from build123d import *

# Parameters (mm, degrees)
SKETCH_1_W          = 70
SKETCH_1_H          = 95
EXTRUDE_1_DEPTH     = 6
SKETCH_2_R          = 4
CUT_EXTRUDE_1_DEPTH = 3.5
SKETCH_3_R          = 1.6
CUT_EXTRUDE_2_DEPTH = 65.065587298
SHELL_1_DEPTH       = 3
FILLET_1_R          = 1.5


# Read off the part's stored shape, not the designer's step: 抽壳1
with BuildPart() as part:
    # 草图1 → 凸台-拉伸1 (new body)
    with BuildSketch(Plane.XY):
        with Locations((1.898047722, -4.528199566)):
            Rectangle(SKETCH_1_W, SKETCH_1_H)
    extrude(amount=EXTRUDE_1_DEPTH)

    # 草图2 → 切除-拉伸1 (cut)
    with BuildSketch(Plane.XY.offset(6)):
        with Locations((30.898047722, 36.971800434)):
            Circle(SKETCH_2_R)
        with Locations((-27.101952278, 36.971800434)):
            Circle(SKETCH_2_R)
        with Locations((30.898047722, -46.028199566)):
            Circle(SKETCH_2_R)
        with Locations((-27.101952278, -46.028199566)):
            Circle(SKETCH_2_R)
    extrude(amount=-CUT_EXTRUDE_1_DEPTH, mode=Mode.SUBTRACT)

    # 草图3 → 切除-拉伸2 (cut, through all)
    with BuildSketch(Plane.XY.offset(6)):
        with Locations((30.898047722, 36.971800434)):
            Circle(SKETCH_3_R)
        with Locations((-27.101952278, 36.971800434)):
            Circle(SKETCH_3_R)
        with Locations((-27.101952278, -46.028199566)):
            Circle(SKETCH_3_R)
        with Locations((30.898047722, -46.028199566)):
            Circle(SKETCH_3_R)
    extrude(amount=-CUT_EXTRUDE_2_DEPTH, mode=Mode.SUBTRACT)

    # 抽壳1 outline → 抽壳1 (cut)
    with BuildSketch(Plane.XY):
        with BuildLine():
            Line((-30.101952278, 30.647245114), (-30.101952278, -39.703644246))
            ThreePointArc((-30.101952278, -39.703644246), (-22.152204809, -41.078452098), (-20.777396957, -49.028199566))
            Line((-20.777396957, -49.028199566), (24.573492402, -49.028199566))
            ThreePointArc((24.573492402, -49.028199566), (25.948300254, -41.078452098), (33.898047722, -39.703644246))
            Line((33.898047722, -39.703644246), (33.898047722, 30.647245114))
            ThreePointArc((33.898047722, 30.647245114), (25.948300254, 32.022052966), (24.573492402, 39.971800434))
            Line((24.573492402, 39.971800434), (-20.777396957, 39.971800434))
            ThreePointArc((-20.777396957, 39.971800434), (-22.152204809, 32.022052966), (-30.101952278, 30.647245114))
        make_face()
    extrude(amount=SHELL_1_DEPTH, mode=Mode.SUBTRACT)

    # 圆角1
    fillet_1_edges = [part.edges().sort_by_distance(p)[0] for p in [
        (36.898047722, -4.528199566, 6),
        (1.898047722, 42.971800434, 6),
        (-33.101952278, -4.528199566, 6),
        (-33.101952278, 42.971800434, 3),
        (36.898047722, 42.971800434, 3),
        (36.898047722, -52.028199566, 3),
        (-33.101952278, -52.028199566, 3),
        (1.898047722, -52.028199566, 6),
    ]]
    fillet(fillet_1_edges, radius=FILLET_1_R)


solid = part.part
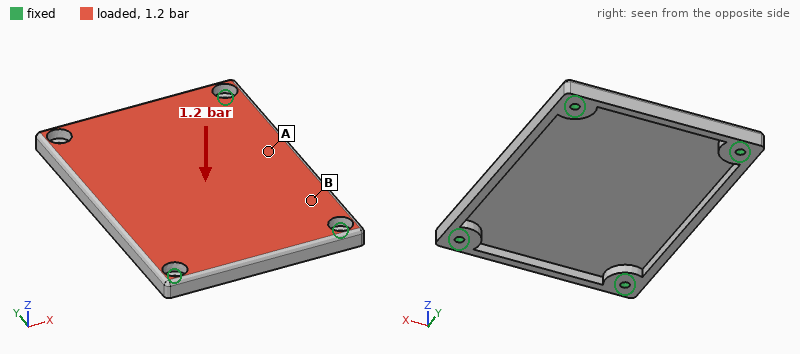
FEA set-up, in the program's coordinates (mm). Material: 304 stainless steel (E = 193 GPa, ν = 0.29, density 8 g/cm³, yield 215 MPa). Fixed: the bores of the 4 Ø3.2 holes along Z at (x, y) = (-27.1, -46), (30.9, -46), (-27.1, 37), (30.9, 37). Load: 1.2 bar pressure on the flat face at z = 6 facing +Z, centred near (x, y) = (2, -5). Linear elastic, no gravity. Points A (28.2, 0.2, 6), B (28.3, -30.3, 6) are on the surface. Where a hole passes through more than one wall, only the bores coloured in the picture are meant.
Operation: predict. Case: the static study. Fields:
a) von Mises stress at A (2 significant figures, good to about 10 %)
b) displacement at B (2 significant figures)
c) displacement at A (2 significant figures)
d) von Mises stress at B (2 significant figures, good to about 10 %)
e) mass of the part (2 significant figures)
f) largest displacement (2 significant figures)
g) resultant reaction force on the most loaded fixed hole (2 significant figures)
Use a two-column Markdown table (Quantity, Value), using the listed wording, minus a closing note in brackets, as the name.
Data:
| Quantity | Value |
|---|---|
| von Mises stress at A | 17 MPa |
| displacement at B | 10 µm |
| displacement at A | 22 µm |
| von Mises stress at B | 8.3 MPa |
| mass of the part | 180 g |
| largest displacement | 34 µm |
| resultant reaction force on the most loaded fixed hole | 450 N |
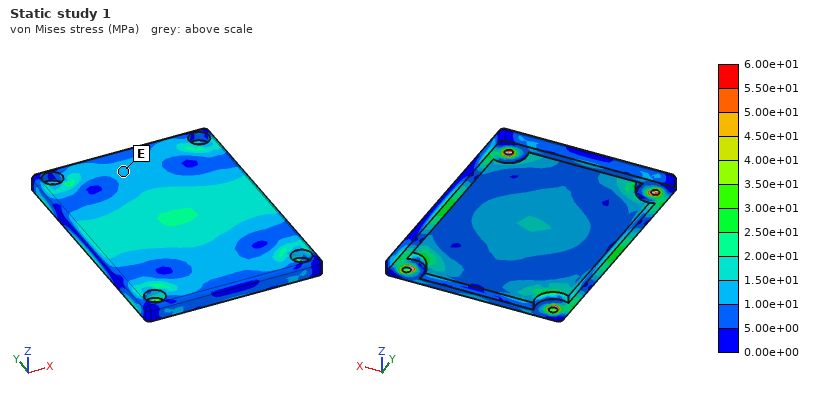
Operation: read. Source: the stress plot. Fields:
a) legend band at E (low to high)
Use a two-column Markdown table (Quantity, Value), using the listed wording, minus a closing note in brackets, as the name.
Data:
| Quantity | Value |
|---|---|
| legend band at E | 1.00e+01 to 1.50e+01 MPa |
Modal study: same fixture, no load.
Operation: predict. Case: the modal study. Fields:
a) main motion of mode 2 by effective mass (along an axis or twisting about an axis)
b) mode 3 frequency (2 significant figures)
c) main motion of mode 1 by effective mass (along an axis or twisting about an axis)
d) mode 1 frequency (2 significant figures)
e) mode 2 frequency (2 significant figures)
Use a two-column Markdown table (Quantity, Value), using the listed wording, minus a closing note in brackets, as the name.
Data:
| Quantity | Value |
|---|---|
| main motion of mode 2 by effective mass | twisting about Y |
| mode 3 frequency | 4900 Hz |
| main motion of mode 1 by effective mass | along Z |
| mode 1 frequency | 2300 Hz |
| mode 2 frequency | 3500 Hz |
